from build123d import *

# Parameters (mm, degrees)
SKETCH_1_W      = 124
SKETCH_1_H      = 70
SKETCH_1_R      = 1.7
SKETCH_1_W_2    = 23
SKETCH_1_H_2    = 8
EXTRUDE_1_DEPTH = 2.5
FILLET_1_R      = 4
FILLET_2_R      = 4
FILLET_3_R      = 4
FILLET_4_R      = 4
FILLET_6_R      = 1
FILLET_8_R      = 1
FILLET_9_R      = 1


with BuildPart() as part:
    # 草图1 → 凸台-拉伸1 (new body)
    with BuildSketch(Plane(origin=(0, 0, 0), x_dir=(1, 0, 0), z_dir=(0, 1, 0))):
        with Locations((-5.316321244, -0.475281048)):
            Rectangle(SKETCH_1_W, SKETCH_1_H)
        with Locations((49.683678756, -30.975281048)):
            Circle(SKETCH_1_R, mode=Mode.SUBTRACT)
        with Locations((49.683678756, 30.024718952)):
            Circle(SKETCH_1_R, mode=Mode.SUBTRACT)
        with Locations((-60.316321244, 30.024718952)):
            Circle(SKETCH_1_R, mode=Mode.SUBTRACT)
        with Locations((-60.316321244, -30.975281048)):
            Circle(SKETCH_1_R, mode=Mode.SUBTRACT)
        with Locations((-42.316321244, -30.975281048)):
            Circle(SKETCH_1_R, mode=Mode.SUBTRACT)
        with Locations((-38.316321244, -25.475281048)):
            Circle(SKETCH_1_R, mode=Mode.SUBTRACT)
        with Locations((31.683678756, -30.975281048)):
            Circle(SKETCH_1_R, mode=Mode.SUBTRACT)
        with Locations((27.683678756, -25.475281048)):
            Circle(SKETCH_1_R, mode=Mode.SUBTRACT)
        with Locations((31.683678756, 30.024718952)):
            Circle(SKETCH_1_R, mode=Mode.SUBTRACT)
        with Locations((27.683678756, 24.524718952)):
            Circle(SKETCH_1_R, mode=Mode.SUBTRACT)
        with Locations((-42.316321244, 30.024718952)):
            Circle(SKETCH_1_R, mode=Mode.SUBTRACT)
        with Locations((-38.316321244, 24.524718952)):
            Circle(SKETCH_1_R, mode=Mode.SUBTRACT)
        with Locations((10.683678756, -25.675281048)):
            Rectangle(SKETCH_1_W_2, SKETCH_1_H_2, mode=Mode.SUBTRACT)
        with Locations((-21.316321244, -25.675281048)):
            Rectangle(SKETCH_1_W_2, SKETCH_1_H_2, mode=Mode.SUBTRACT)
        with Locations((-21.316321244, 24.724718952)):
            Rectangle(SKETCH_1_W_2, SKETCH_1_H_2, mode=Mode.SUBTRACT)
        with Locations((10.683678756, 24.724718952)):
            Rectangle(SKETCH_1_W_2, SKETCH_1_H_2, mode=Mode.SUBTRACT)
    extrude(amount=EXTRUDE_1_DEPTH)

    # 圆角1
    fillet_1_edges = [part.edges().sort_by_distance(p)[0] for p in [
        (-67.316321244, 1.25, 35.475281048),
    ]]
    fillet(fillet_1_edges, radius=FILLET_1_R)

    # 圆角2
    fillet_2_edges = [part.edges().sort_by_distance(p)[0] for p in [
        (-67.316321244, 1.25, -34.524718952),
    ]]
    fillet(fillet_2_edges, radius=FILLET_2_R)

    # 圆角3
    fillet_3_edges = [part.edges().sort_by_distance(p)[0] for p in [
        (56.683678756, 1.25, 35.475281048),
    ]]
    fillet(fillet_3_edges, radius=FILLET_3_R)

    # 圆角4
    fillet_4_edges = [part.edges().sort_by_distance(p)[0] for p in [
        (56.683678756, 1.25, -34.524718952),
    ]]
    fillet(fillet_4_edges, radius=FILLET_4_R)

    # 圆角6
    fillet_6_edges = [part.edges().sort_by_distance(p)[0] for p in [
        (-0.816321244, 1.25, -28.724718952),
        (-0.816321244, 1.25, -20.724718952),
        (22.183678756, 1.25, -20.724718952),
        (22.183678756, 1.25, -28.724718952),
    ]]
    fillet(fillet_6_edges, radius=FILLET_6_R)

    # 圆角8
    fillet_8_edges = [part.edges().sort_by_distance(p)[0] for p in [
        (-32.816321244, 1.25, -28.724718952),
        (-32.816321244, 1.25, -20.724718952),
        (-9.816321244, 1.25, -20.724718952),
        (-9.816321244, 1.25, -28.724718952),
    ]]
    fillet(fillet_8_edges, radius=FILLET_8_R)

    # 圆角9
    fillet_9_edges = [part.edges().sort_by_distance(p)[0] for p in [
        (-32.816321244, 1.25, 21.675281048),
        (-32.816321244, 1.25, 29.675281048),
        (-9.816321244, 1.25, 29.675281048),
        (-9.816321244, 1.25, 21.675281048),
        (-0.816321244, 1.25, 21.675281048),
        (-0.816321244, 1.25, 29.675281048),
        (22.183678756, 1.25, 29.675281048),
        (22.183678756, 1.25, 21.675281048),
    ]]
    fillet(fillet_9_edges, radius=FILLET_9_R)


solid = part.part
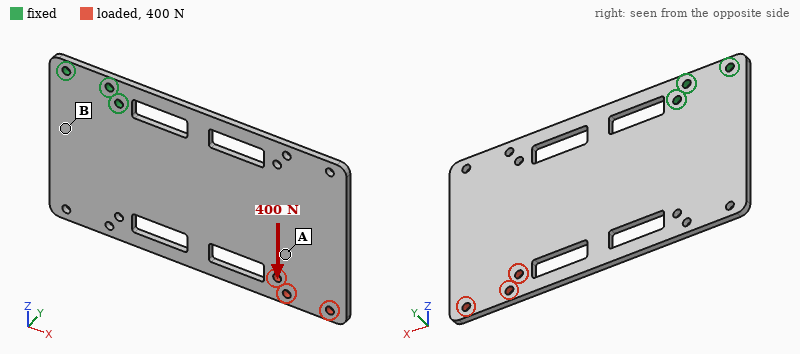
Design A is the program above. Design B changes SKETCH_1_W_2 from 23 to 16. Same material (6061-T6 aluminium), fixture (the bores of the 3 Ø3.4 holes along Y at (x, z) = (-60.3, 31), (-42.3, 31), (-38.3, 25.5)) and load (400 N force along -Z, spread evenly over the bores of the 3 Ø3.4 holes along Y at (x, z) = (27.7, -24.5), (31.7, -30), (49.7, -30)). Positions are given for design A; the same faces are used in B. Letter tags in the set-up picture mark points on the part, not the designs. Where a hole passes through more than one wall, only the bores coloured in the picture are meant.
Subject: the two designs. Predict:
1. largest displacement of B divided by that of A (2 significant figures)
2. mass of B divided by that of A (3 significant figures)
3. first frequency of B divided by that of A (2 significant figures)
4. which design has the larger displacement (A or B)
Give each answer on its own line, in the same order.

0.91
1.03
1.0
A
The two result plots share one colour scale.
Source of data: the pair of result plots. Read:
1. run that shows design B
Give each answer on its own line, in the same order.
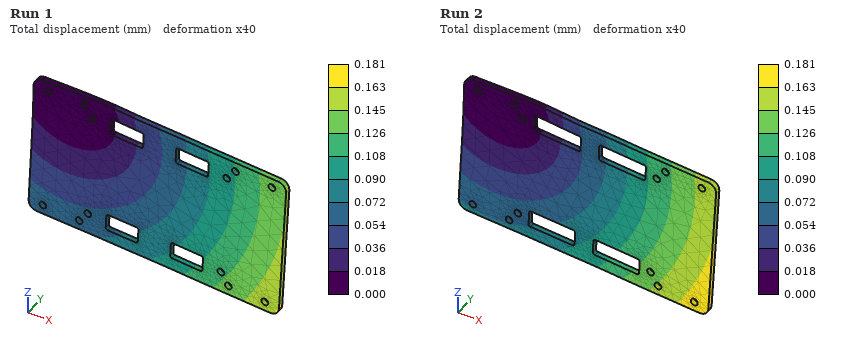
Run 1
